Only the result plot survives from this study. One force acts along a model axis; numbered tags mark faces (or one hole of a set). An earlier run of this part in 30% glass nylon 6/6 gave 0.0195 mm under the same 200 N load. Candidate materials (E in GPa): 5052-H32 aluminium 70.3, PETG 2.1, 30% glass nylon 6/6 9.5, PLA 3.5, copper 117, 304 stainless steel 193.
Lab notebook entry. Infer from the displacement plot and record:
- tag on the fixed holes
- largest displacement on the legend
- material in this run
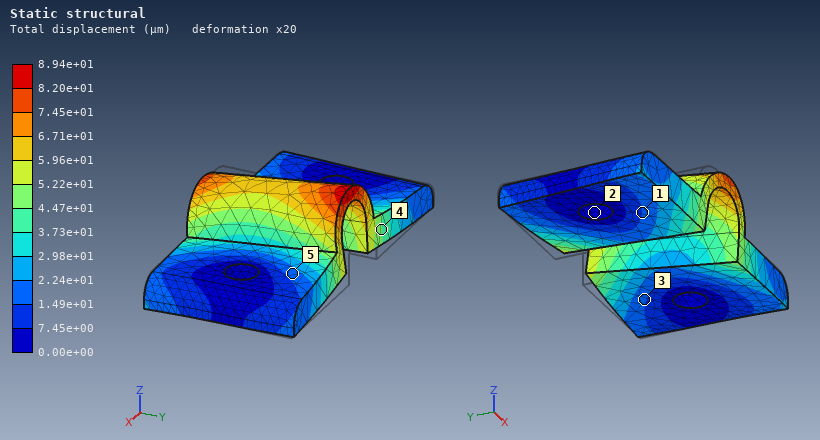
2
8.94e+01 µm
PETG
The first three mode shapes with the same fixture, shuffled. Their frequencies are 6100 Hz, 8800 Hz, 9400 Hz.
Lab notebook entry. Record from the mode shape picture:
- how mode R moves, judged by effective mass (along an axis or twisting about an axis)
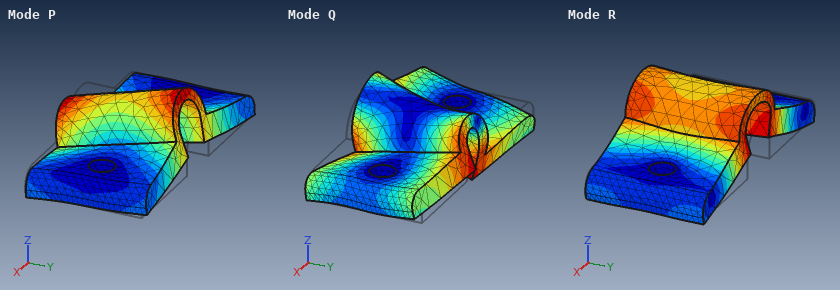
along Z
